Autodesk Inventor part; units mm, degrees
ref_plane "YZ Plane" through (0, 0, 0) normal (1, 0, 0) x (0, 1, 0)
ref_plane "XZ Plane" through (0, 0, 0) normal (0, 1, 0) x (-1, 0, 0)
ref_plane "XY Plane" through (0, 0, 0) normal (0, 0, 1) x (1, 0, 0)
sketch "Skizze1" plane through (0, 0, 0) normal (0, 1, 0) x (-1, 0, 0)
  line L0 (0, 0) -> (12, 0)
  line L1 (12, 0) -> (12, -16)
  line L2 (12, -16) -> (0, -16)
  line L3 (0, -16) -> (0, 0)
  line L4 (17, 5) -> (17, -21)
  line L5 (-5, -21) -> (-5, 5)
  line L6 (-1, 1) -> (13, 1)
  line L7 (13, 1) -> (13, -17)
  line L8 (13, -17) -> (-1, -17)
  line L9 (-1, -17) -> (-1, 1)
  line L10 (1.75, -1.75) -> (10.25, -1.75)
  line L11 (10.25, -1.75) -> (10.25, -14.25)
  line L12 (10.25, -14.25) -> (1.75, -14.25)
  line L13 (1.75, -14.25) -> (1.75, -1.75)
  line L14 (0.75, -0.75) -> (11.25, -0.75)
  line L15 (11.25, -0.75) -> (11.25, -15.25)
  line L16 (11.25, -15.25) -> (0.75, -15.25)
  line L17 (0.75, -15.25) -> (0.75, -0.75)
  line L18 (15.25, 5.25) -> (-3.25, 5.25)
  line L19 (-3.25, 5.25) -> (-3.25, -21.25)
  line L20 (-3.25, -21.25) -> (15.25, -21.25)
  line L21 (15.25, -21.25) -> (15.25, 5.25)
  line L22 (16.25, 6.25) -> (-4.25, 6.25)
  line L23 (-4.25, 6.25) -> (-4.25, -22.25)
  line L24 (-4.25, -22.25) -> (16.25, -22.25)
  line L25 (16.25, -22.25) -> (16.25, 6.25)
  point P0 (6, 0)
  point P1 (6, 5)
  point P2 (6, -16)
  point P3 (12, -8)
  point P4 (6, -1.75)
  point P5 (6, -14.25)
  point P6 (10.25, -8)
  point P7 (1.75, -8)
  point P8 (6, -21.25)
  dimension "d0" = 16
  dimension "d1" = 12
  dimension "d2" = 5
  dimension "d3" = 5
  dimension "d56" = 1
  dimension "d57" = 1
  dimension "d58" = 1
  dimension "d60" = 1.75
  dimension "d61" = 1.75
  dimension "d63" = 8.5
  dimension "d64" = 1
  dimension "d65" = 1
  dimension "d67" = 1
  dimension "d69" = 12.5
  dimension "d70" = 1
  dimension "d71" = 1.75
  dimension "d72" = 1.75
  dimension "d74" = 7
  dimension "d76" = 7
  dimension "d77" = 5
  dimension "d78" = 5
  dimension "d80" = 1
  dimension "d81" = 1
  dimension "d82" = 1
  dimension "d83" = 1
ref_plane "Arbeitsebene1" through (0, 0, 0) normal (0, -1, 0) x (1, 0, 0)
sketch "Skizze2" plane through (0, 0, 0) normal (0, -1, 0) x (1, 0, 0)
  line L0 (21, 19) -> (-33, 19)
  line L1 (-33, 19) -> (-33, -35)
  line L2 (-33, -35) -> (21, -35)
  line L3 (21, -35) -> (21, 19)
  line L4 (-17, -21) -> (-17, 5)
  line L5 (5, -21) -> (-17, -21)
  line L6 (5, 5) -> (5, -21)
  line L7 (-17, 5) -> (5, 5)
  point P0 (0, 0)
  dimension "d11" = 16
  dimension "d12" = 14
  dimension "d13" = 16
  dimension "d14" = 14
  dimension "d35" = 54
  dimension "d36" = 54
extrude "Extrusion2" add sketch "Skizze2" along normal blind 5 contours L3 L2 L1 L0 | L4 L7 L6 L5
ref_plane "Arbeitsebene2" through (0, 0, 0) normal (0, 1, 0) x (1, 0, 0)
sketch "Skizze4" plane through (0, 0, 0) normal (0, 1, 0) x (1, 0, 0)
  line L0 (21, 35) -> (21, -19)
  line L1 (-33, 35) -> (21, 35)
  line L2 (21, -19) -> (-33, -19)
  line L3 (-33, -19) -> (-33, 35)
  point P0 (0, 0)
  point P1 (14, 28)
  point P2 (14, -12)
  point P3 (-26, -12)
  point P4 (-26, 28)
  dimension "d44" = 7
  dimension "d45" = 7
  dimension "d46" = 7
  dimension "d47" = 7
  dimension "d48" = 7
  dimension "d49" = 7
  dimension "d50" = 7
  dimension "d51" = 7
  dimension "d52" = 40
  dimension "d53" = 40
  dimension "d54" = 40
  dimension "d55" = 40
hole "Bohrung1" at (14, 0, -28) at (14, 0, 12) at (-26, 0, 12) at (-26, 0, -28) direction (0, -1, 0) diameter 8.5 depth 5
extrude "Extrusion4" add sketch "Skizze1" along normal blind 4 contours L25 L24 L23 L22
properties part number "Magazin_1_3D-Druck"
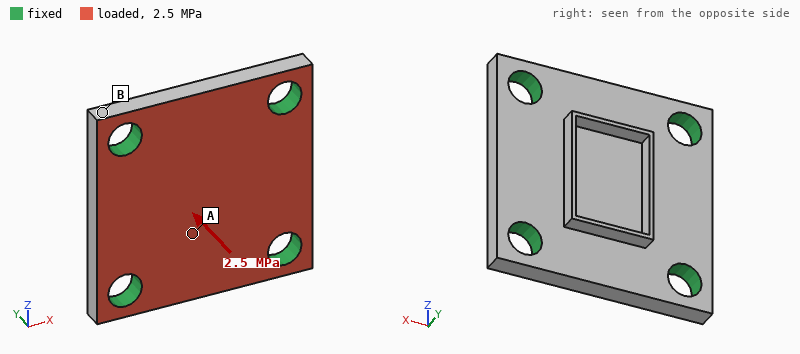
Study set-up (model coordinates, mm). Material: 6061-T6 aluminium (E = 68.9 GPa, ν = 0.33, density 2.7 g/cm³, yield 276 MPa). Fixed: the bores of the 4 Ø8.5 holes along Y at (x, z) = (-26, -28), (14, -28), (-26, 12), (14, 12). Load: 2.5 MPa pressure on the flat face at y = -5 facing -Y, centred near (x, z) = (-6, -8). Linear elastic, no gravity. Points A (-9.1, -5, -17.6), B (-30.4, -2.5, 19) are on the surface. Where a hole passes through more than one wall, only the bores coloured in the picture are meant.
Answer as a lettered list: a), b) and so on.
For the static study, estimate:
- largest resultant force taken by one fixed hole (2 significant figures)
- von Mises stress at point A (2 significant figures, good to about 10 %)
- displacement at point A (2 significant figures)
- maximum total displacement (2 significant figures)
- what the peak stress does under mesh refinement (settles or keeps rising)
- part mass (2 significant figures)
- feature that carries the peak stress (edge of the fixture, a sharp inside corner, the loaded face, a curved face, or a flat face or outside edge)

a) 1.7 kN
b) 25 MPa
c) 27 µm
d) 33 µm
e) keeps rising
f) 37 g
g) edge of the fixture
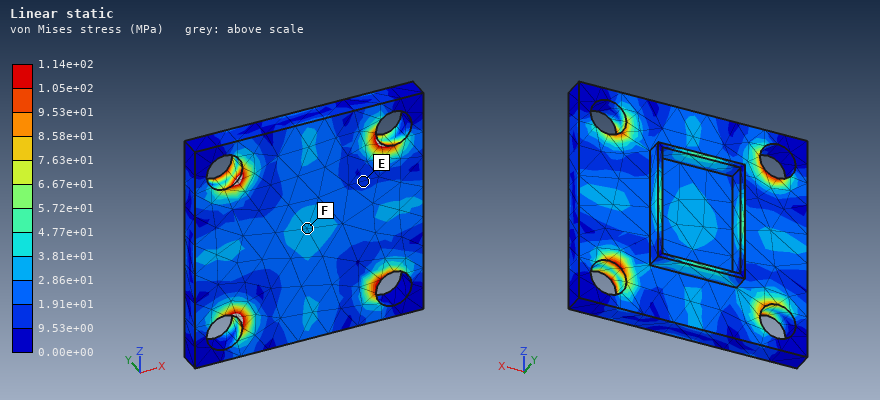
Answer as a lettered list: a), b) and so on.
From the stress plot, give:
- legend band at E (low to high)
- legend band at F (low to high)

a) 9.53e+00 to 1.91e+01 MPa
b) 2.86e+01 to 3.81e+01 MPa
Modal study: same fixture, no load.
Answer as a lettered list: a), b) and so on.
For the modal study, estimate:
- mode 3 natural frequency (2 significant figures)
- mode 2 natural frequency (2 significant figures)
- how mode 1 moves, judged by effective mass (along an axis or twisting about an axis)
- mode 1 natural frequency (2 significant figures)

a) 21 kHz
b) 21 kHz
c) along Y
d) 14 kHz
